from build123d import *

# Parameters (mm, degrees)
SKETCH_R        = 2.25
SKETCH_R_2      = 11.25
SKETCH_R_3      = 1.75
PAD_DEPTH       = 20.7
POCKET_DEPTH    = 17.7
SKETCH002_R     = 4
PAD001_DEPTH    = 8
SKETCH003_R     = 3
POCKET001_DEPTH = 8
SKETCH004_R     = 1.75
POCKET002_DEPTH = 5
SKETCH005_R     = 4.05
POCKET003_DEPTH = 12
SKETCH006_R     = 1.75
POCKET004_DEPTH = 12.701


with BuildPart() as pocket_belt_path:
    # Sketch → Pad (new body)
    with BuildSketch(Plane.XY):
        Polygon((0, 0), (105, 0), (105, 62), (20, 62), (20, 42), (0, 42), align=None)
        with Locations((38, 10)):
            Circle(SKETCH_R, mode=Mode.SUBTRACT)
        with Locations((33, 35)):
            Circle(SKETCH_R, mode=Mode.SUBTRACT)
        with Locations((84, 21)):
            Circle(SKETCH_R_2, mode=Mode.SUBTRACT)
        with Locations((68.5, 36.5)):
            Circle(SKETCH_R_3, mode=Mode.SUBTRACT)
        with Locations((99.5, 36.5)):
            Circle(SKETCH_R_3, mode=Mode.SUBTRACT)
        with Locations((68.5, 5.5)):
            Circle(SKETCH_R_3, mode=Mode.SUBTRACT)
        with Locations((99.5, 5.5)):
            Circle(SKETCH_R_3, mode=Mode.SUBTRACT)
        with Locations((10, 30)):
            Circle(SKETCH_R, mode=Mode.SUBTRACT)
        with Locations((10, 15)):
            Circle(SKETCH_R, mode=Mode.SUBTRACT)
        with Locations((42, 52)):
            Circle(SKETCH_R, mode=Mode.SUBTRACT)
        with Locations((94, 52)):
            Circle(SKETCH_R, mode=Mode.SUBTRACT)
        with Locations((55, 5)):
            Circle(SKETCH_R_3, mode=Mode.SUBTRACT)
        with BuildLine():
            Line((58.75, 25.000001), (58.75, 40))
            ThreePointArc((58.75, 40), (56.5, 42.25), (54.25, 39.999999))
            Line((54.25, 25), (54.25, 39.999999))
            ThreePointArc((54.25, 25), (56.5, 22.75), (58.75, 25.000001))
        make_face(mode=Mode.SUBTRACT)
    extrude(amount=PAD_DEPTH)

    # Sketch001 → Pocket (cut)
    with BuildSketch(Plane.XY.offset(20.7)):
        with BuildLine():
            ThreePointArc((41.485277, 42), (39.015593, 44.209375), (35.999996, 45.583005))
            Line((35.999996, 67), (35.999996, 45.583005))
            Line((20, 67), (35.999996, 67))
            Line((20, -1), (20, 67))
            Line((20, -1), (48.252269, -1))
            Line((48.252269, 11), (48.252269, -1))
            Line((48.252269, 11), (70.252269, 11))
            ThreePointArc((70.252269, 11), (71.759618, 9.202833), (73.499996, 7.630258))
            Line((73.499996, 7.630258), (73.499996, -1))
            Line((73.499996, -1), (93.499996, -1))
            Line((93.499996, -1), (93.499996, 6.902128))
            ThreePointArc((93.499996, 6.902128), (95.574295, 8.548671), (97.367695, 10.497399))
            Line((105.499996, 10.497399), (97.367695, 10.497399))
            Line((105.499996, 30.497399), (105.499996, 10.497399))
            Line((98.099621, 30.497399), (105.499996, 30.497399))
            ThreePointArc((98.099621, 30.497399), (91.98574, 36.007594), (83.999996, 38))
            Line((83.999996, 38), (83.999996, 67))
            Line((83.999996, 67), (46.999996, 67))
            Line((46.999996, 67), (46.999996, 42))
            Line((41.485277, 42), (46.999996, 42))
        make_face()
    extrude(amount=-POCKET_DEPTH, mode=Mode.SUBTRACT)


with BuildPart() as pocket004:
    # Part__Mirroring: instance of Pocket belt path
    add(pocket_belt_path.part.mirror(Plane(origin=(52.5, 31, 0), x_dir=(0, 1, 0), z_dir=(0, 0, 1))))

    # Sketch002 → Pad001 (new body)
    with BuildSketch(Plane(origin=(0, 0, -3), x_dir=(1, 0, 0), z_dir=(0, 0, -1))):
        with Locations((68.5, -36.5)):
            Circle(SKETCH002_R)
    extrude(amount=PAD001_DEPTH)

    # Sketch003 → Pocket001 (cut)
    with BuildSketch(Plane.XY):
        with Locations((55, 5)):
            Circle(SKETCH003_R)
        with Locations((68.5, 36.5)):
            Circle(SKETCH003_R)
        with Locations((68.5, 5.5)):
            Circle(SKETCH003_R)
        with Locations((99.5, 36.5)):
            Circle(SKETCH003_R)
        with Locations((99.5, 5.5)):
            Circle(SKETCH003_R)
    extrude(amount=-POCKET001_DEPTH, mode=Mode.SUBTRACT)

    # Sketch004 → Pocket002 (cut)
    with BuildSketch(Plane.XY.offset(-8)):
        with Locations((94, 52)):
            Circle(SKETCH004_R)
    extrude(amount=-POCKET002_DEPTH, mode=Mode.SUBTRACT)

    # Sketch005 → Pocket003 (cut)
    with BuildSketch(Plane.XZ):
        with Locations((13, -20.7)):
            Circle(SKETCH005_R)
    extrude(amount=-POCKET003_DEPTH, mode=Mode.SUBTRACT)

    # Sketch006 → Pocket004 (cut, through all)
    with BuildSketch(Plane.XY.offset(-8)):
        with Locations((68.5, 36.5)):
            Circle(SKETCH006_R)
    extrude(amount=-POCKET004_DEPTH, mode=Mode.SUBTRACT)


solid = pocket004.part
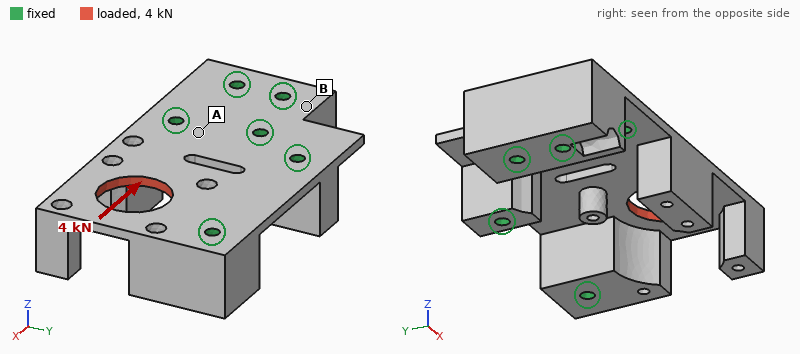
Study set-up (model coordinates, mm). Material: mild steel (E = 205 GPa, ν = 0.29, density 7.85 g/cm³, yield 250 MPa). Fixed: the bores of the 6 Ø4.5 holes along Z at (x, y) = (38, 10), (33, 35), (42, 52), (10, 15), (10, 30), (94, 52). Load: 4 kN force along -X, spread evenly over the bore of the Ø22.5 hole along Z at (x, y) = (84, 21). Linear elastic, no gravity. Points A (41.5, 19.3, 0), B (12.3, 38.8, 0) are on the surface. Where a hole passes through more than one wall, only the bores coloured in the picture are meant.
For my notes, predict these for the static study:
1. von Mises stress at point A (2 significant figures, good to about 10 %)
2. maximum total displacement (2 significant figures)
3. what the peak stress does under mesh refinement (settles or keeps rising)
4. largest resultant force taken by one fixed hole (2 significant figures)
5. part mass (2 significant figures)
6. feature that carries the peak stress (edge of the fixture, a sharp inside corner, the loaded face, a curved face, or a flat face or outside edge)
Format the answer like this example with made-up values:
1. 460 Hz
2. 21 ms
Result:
1. 11 MPa
2. 12 µm
3. keeps rising
4. 1.6 kN
5. 390 g
6. a sharp inside corner
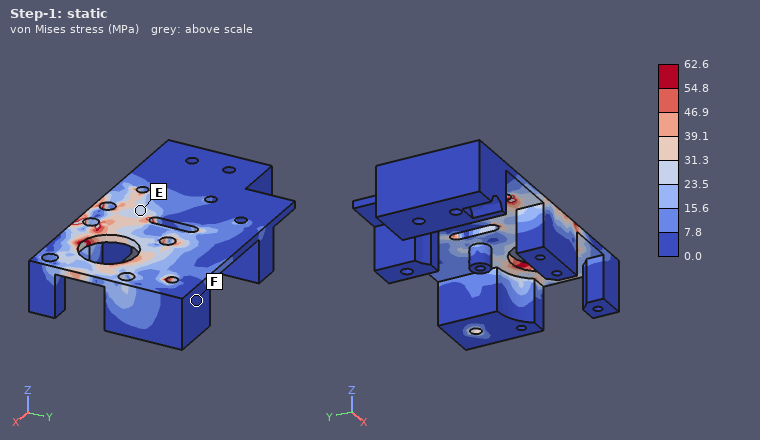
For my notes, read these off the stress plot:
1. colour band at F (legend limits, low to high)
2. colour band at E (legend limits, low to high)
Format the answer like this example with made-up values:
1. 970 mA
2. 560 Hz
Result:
1. 0.0 to 7.8 MPa
2. 23.5 to 31.3 MPa
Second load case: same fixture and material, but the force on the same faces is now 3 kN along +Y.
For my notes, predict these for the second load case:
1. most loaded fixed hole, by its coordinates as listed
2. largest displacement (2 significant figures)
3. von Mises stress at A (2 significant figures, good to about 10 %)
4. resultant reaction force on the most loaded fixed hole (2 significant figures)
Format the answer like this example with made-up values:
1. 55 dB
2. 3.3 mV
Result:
1. (94, 52)
2. 11 µm
3. 8.8 MPa
4. 2.2 kN
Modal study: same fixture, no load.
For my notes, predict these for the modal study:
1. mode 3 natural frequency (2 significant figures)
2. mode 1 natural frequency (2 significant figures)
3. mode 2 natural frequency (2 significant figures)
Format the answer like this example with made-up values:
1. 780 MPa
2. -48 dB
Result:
1. 3700 Hz
2. 1200 Hz
3. 2200 Hz
